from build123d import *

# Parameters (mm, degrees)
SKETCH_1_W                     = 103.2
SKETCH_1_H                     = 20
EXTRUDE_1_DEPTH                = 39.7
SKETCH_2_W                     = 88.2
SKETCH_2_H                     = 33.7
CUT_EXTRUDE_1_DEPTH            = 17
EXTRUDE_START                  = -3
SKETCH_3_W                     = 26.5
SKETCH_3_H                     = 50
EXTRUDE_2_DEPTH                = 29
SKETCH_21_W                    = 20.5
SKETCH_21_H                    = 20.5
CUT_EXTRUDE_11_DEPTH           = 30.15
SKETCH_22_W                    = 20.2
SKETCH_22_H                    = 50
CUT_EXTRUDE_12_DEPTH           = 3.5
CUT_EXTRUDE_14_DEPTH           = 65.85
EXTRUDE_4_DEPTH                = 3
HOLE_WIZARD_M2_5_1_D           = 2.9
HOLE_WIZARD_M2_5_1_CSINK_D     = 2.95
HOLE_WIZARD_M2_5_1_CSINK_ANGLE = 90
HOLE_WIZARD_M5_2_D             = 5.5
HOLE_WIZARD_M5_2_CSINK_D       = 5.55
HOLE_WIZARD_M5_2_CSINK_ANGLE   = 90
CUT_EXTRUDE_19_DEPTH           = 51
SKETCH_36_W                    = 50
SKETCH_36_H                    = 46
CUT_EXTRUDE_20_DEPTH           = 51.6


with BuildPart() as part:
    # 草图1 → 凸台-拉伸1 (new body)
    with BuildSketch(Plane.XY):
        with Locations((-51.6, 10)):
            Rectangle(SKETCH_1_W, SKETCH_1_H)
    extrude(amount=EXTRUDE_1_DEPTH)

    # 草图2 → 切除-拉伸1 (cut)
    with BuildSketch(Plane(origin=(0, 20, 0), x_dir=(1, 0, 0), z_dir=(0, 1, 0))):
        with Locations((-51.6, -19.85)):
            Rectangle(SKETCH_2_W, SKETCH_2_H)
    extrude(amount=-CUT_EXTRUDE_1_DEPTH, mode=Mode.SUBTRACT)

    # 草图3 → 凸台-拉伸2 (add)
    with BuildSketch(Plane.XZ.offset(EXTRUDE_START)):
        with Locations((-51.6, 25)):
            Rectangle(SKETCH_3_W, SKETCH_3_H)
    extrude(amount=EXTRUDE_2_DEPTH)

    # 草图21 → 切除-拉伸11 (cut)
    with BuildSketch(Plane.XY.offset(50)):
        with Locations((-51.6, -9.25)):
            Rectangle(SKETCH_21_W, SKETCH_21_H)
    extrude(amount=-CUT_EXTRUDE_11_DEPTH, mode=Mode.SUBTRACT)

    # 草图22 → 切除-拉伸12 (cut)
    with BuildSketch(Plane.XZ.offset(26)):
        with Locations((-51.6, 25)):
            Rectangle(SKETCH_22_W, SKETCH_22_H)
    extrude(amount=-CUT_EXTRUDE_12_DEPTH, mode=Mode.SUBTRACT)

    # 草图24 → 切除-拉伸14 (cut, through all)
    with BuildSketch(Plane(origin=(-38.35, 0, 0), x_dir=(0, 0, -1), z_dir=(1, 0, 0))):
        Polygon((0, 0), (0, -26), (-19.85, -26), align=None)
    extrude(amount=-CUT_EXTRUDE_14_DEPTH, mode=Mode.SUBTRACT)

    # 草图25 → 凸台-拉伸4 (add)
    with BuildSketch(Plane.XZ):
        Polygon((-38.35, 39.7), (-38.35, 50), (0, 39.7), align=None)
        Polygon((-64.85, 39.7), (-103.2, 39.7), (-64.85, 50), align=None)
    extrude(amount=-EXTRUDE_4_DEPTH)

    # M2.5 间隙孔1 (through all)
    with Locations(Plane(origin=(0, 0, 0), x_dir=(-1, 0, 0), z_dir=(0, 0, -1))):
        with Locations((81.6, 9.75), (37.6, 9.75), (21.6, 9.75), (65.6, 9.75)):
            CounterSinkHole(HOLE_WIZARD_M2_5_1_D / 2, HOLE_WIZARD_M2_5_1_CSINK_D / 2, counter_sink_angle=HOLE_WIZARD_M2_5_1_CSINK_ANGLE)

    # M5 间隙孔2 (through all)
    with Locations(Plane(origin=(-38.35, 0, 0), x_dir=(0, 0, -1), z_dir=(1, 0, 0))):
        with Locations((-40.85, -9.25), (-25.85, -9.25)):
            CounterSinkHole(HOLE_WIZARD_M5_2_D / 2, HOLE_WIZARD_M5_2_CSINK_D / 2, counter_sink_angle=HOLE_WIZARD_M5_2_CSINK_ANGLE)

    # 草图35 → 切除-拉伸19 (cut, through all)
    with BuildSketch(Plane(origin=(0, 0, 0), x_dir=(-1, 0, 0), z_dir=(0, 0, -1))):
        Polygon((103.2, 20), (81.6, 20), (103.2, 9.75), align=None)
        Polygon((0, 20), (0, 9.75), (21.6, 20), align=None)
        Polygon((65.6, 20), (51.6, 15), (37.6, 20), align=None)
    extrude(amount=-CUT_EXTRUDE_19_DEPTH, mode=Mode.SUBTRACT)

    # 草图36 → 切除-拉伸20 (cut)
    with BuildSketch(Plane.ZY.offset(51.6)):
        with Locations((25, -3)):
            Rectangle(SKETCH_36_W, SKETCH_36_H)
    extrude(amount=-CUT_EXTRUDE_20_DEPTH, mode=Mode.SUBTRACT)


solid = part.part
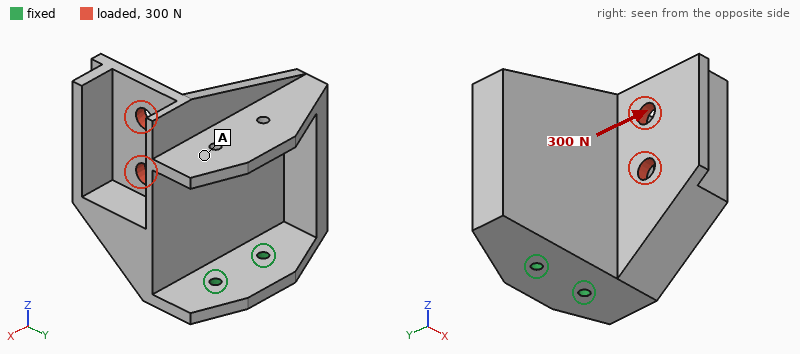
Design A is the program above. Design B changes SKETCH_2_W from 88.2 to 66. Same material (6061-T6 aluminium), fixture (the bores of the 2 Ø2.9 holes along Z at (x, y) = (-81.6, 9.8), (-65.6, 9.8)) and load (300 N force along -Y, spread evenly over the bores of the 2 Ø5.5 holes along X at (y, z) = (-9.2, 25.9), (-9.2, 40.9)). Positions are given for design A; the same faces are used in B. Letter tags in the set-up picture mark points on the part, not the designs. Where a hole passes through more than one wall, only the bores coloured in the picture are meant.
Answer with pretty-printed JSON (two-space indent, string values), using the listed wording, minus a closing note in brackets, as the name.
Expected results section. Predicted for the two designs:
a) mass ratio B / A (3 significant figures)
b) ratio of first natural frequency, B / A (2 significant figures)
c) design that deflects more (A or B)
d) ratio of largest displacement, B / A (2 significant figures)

{
  "mass ratio B / A": "1.24",
  "ratio of first natural frequency, B / A": "1.3",
  "design that deflects more": "A",
  "ratio of largest displacement, B / A": "0.51"
}
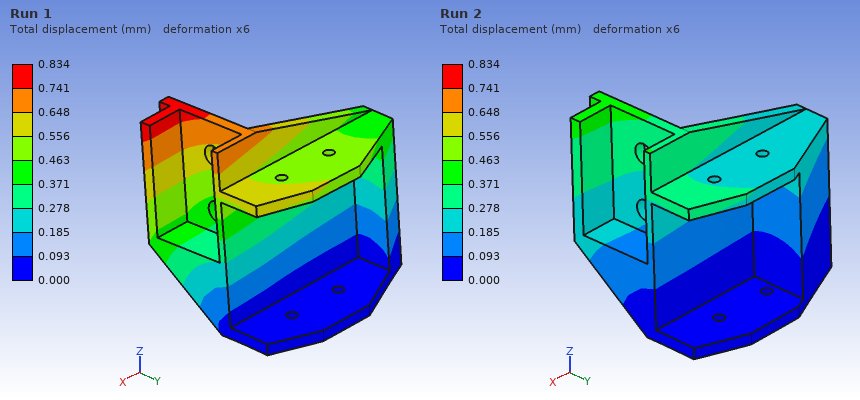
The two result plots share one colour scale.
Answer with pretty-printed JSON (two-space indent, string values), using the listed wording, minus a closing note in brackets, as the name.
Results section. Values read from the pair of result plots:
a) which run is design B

{
  "which run is design B": "Run 2"
}
